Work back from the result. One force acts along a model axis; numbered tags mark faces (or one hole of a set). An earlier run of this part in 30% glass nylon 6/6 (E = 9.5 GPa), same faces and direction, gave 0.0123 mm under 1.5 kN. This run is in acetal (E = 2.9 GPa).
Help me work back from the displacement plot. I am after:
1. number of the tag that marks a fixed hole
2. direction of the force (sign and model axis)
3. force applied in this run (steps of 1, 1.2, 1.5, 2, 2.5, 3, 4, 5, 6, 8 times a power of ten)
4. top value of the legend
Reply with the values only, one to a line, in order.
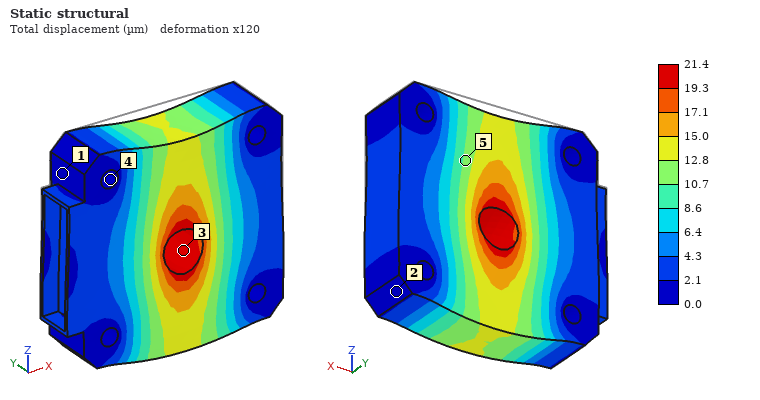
4
-Z
800 N
21.4 µm
